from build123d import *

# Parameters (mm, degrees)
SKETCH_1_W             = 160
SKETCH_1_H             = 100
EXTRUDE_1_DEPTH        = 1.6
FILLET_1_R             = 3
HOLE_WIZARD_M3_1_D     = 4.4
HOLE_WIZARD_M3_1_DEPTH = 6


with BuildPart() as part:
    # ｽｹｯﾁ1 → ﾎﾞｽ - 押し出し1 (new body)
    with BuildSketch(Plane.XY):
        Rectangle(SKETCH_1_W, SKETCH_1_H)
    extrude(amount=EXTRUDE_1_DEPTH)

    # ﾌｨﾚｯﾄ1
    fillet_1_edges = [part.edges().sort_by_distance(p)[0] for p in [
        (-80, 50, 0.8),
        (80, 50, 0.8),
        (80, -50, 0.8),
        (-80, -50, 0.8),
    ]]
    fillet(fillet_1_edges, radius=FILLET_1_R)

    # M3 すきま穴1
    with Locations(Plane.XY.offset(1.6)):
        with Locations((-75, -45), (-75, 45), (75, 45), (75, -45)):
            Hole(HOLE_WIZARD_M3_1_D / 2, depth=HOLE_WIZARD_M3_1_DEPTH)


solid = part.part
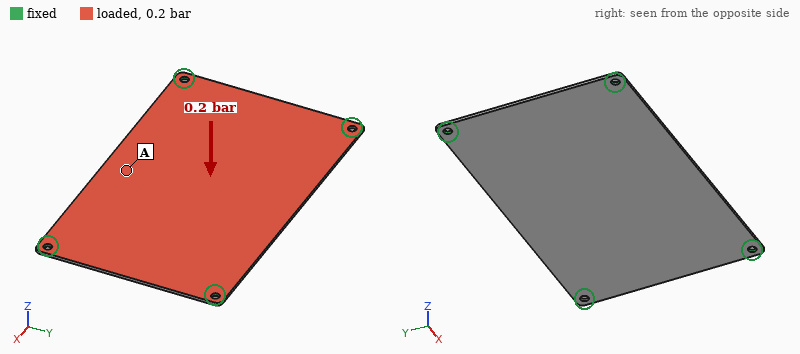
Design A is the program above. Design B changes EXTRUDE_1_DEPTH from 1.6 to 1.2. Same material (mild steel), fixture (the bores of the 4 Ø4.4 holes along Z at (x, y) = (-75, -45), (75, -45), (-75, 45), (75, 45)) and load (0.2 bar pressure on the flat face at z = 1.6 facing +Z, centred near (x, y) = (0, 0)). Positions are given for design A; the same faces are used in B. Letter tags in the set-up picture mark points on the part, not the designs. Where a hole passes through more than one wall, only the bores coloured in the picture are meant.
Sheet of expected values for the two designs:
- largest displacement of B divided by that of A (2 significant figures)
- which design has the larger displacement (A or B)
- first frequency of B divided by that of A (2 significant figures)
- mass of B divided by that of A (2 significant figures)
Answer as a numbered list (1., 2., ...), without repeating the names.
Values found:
1. 2.3
2. B
3. 0.75
4. 0.75
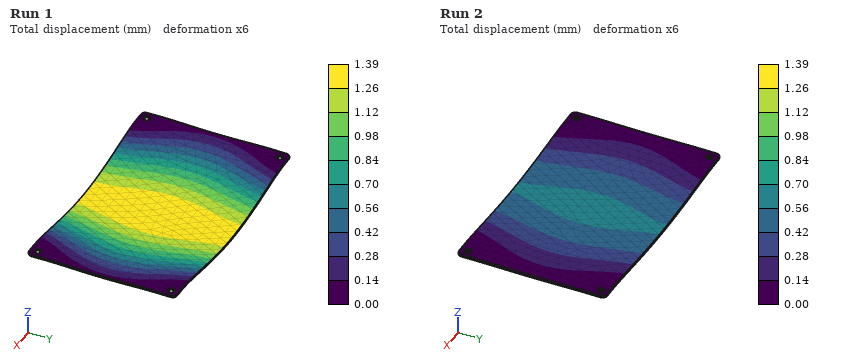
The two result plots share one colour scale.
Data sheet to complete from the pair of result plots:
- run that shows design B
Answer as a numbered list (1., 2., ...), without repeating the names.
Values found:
1. Run 1
